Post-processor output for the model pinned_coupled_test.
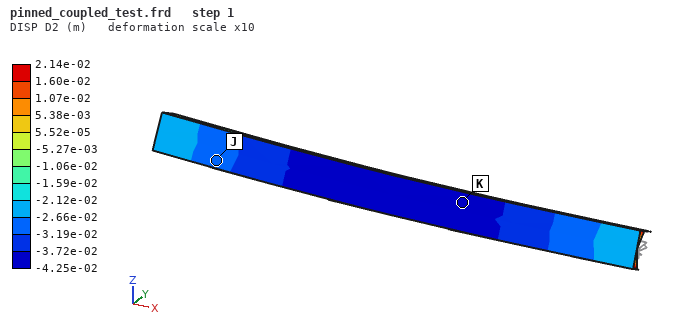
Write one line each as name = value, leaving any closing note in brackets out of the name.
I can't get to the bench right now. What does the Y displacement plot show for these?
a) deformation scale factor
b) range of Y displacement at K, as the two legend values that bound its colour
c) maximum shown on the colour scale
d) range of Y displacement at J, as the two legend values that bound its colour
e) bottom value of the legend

deformation scale factor = 10
range of Y displacement at K, as the two legend values that bound its colour = -4.25e-02 to -3.72e-02 m
maximum shown on the colour scale = 2.14e-02 m
range of Y displacement at J, as the two legend values that bound its colour = -3.19e-02 to -2.66e-02 m
bottom value of the legend = -4.25e-02 m
